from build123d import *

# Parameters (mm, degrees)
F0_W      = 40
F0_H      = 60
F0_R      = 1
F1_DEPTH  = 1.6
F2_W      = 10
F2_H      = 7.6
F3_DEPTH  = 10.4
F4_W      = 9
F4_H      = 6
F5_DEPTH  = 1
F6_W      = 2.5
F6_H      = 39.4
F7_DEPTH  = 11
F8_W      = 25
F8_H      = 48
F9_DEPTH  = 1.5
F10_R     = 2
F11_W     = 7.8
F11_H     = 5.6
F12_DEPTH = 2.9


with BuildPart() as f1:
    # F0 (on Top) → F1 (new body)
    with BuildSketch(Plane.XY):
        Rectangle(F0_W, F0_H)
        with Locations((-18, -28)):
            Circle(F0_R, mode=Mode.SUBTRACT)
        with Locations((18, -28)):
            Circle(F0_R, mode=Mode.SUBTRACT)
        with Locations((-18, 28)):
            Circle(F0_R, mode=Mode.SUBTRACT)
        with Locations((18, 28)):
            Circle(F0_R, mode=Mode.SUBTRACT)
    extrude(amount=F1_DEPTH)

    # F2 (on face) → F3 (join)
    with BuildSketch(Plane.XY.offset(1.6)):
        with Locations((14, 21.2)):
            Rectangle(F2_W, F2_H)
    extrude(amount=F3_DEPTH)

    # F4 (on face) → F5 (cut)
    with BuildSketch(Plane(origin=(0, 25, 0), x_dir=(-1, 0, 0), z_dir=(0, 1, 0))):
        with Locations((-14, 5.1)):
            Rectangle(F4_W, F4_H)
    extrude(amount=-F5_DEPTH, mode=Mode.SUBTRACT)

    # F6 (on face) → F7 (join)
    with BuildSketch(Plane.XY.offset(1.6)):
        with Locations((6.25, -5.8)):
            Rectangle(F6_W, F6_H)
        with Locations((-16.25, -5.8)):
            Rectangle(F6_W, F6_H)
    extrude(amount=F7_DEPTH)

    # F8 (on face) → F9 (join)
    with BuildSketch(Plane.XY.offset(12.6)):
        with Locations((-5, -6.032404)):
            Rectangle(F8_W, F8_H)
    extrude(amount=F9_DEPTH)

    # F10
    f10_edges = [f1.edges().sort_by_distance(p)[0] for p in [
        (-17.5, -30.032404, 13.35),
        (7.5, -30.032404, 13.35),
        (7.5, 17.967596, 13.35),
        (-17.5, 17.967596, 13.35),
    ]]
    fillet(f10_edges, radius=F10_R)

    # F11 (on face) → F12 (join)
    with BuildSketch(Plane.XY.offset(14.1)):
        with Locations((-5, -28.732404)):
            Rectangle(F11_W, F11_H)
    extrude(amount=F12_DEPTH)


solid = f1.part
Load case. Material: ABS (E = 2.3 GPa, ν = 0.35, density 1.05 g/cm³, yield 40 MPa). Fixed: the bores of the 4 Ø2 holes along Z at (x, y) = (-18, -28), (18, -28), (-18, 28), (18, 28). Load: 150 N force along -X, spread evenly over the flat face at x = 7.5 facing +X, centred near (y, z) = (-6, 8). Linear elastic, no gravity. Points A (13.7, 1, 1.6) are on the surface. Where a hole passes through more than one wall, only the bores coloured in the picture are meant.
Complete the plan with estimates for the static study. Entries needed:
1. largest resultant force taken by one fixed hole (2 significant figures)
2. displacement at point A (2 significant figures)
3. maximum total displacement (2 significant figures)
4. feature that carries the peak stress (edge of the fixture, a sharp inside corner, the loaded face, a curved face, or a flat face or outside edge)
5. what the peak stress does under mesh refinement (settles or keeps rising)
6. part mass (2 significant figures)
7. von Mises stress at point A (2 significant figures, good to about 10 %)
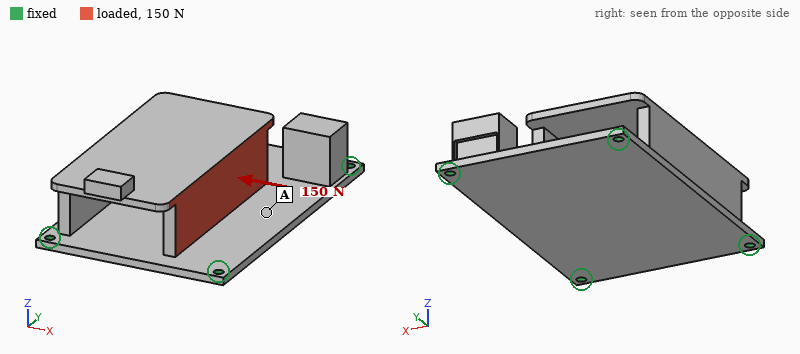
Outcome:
63 N
0.41 mm
0.57 mm
edge of the fixture
keeps rising
9.1 g
2.9 MPa
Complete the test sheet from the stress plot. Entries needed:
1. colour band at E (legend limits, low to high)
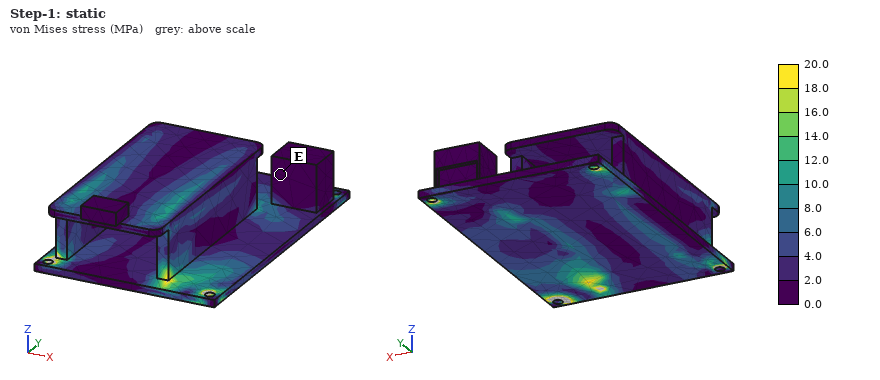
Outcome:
0.0 to 2.0 MPa
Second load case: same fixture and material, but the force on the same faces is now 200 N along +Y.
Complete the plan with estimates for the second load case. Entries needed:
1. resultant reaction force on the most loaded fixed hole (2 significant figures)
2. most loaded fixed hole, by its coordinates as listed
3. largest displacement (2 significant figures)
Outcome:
64 N
(18, -28)
0.77 mm
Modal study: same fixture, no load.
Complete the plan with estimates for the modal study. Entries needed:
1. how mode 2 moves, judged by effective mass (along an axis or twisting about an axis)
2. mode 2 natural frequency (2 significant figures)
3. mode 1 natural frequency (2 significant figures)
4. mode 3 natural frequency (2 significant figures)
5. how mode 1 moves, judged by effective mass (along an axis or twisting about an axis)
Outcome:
along X
990 Hz
670 Hz
1500 Hz
along Z
